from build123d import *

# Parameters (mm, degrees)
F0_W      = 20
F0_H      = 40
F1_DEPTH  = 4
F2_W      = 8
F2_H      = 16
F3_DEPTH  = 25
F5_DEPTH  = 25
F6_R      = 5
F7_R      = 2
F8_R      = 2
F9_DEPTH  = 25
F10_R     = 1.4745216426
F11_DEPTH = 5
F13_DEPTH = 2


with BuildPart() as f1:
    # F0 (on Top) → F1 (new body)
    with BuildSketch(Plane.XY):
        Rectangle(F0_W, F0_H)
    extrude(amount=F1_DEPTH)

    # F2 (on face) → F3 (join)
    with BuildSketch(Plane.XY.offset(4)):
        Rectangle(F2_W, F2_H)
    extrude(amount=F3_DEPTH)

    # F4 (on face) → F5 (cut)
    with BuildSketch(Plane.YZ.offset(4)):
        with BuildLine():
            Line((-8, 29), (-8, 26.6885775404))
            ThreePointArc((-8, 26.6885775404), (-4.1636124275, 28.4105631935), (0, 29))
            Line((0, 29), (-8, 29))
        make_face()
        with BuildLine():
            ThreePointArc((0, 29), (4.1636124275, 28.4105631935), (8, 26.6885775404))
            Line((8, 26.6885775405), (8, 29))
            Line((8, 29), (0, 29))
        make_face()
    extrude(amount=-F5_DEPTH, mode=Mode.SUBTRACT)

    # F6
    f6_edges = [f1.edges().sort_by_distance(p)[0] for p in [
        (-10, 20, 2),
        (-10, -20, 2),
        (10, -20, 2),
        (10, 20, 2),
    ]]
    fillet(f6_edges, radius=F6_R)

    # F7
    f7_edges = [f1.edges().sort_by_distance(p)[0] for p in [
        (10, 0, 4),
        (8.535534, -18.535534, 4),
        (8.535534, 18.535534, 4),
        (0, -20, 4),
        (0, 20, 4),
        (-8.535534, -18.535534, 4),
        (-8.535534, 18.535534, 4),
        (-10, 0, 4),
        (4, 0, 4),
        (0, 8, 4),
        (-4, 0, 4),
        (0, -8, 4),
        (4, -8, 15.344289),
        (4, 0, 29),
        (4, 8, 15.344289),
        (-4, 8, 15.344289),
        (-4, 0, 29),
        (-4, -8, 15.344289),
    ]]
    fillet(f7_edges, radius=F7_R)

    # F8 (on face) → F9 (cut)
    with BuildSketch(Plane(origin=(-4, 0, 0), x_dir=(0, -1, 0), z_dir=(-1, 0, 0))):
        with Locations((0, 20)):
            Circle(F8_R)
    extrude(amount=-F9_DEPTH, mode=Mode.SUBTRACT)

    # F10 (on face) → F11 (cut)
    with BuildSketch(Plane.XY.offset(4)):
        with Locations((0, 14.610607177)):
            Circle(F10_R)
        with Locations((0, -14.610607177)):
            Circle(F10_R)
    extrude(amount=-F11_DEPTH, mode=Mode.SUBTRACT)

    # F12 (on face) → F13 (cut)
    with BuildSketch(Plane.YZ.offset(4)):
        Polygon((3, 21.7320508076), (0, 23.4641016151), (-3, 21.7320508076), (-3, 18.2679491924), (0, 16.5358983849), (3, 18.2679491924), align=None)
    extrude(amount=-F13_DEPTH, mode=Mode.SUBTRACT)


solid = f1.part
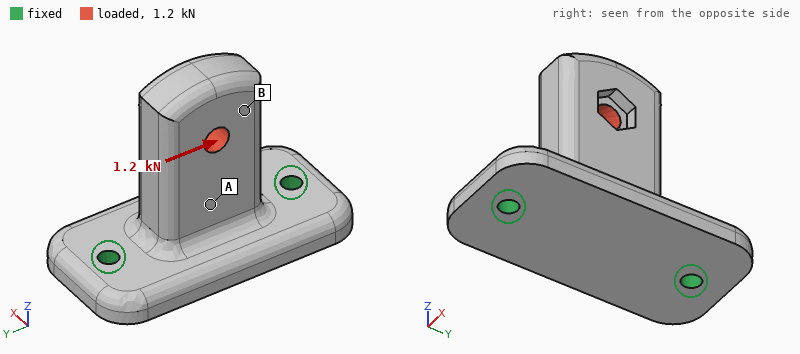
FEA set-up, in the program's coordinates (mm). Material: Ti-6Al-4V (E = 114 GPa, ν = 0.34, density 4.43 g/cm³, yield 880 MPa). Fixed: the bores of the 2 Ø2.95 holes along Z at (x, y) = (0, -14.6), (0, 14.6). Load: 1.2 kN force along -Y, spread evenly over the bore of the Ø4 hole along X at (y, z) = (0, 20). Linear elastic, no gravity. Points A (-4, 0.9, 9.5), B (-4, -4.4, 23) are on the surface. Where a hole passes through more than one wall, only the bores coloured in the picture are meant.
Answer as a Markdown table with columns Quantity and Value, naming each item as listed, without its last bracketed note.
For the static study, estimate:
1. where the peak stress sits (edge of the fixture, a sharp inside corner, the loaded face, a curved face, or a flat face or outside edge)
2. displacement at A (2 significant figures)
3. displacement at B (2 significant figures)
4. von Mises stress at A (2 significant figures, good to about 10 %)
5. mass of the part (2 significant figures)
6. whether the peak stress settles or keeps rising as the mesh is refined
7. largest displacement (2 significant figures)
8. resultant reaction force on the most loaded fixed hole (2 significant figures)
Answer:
| Quantity | Value |
|---|---|
| where the peak stress sits | edge of the fixture |
| displacement at A | 8.0 µm |
| displacement at B | 29 µm |
| von Mises stress at A | 28 MPa |
| mass of the part | 26 g |
| whether the peak stress settles or keeps rising as the mesh is refined | keeps rising |
| largest displacement | 35 µm |
| resultant reaction force on the most loaded fixed hole | 1.1 kN |
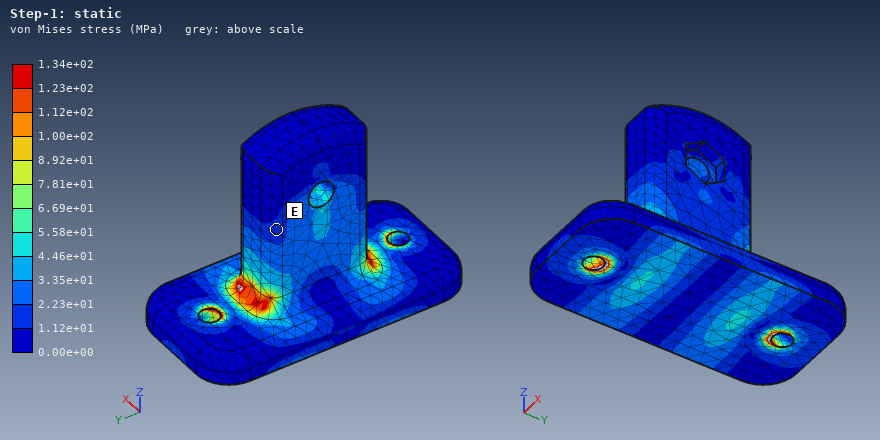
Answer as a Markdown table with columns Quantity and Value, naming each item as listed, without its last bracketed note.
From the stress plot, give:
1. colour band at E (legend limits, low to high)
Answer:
| Quantity | Value |
|---|---|
| colour band at E | 1.12e+01 to 2.23e+01 MPa |
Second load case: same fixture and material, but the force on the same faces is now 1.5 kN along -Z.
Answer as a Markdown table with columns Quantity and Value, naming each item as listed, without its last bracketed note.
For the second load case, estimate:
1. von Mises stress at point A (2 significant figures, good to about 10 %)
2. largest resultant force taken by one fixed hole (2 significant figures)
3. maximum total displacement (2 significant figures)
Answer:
| Quantity | Value |
|---|---|
| von Mises stress at point A | 14 MPa |
| largest resultant force taken by one fixed hole | 800 N |
| maximum total displacement | 20 µm |
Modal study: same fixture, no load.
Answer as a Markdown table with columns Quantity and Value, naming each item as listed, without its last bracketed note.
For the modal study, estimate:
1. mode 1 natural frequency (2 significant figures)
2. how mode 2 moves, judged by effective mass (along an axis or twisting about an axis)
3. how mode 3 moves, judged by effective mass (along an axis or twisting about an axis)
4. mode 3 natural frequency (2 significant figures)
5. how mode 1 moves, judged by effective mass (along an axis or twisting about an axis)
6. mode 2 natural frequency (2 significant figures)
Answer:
| Quantity | Value |
|---|---|
| mode 1 natural frequency | 4700 Hz |
| how mode 2 moves, judged by effective mass | along Y |
| how mode 3 moves, judged by effective mass | along Z |
| mode 3 natural frequency | 15 kHz |
| how mode 1 moves, judged by effective mass | along X |
| mode 2 natural frequency | 11 kHz |
